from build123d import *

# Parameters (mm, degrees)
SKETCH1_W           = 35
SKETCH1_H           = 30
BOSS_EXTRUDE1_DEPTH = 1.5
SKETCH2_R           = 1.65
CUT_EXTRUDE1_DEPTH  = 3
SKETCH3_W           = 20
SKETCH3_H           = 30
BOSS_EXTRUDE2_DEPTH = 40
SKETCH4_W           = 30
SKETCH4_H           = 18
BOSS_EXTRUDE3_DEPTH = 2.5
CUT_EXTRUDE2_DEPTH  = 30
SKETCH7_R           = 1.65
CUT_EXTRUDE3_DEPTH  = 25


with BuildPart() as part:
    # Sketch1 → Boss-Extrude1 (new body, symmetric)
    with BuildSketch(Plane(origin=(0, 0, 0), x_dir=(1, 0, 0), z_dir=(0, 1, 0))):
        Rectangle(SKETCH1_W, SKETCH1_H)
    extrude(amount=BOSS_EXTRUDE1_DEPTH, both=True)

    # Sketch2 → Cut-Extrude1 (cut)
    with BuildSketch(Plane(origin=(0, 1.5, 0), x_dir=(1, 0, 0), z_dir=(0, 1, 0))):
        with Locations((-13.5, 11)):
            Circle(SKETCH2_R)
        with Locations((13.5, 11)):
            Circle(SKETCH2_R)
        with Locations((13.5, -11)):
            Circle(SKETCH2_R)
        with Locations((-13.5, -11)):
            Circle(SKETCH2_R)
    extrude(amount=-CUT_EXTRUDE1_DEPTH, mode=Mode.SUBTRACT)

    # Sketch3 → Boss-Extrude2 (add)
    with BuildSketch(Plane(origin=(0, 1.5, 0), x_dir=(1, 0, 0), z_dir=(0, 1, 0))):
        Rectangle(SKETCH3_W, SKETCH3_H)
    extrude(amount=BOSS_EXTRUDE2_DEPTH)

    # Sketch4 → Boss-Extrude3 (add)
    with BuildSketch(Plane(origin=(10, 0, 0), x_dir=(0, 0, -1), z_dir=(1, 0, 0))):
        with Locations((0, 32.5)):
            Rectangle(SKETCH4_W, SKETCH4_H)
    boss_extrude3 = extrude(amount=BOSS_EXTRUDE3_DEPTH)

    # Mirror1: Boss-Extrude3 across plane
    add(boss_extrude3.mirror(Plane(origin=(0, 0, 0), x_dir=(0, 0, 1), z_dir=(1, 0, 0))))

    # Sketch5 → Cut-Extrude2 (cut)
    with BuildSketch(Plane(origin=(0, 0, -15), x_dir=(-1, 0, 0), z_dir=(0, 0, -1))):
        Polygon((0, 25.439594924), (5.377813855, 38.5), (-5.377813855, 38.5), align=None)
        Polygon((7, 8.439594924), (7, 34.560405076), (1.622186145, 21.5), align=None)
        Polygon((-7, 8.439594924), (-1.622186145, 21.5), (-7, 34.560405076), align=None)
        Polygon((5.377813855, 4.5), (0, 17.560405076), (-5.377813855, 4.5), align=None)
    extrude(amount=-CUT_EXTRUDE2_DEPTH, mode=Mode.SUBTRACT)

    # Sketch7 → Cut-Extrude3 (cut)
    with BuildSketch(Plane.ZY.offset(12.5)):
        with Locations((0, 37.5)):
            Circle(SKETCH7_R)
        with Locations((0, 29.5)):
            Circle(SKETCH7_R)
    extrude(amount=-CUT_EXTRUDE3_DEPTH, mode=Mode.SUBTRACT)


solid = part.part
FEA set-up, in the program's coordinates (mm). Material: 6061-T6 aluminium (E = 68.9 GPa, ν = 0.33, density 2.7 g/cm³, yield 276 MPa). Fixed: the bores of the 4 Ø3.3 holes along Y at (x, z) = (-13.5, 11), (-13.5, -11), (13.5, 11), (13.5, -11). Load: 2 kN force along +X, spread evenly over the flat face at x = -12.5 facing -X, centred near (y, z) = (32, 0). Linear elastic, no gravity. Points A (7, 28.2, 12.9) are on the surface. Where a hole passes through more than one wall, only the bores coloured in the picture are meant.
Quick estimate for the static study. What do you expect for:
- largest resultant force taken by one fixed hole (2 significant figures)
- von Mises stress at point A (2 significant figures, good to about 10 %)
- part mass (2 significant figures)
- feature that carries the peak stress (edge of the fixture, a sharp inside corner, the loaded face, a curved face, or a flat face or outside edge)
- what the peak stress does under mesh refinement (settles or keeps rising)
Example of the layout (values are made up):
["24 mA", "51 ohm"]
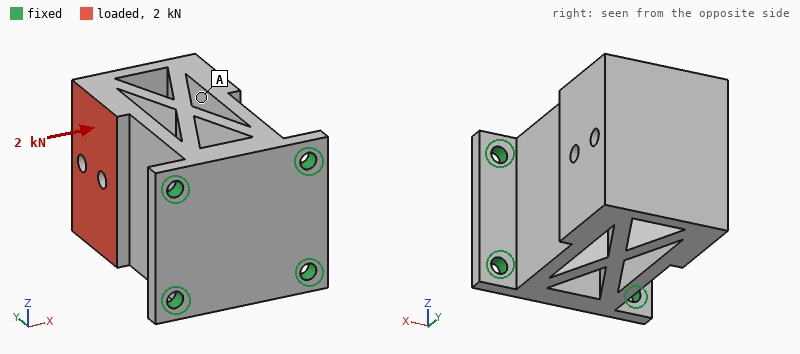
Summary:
["1.5 kN", "22 MPa", "57 g", "edge of the fixture", "keeps rising"]
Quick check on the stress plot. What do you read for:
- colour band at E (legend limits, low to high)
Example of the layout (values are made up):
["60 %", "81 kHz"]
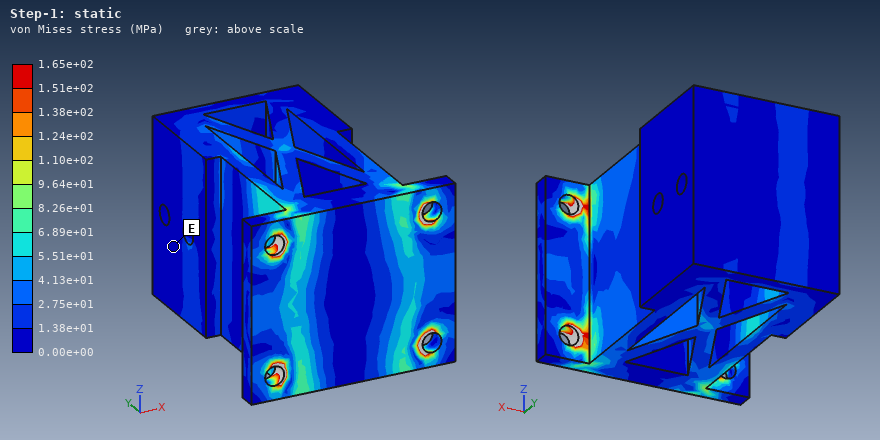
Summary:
["0.00e+00 to 1.38e+01 MPa"]
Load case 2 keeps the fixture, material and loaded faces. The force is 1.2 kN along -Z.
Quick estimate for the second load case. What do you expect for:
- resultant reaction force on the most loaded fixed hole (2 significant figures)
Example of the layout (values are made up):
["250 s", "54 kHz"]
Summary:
["1.0 kN"]
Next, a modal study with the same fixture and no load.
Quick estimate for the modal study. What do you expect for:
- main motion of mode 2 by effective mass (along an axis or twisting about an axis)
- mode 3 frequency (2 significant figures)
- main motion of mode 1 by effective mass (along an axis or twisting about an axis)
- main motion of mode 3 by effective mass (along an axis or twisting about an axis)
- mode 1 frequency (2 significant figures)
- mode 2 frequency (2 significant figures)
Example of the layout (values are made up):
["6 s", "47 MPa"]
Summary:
["along Z", "9200 Hz", "along X", "twisting about Y", "4300 Hz", "4600 Hz"]
